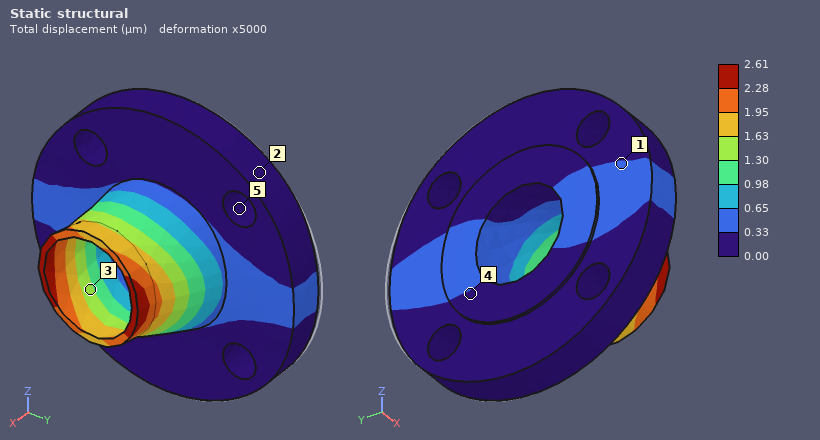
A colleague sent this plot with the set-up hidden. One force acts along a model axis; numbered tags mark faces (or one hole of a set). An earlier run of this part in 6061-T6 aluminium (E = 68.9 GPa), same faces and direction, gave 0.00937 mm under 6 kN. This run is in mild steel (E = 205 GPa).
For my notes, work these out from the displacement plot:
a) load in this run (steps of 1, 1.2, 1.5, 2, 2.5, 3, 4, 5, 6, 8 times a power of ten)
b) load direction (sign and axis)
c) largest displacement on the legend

5 kN
-Y
2.61 µm
